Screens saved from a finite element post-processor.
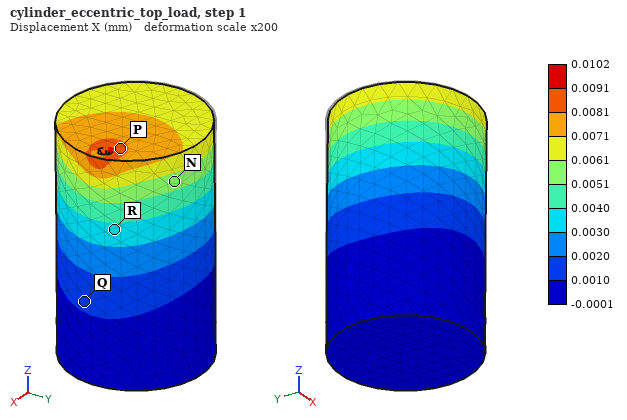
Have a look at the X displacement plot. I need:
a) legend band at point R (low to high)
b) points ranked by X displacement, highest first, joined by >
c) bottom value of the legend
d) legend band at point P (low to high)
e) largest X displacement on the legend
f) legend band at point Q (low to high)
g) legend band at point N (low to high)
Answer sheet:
0.0030 to 0.0040 mm
P > N > R > Q
-0.0001 mm
0.0081 to 0.0091 mm
0.0102 mm
0.0010 to 0.0020 mm
0.0051 to 0.0061 mm
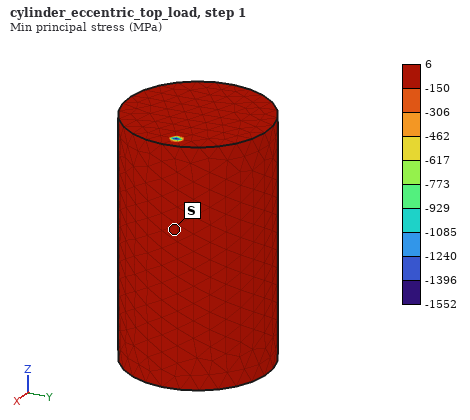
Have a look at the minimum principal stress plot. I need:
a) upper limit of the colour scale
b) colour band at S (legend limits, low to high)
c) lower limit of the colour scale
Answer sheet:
6 MPa
-150 to 6 MPa
-1552 MPa
